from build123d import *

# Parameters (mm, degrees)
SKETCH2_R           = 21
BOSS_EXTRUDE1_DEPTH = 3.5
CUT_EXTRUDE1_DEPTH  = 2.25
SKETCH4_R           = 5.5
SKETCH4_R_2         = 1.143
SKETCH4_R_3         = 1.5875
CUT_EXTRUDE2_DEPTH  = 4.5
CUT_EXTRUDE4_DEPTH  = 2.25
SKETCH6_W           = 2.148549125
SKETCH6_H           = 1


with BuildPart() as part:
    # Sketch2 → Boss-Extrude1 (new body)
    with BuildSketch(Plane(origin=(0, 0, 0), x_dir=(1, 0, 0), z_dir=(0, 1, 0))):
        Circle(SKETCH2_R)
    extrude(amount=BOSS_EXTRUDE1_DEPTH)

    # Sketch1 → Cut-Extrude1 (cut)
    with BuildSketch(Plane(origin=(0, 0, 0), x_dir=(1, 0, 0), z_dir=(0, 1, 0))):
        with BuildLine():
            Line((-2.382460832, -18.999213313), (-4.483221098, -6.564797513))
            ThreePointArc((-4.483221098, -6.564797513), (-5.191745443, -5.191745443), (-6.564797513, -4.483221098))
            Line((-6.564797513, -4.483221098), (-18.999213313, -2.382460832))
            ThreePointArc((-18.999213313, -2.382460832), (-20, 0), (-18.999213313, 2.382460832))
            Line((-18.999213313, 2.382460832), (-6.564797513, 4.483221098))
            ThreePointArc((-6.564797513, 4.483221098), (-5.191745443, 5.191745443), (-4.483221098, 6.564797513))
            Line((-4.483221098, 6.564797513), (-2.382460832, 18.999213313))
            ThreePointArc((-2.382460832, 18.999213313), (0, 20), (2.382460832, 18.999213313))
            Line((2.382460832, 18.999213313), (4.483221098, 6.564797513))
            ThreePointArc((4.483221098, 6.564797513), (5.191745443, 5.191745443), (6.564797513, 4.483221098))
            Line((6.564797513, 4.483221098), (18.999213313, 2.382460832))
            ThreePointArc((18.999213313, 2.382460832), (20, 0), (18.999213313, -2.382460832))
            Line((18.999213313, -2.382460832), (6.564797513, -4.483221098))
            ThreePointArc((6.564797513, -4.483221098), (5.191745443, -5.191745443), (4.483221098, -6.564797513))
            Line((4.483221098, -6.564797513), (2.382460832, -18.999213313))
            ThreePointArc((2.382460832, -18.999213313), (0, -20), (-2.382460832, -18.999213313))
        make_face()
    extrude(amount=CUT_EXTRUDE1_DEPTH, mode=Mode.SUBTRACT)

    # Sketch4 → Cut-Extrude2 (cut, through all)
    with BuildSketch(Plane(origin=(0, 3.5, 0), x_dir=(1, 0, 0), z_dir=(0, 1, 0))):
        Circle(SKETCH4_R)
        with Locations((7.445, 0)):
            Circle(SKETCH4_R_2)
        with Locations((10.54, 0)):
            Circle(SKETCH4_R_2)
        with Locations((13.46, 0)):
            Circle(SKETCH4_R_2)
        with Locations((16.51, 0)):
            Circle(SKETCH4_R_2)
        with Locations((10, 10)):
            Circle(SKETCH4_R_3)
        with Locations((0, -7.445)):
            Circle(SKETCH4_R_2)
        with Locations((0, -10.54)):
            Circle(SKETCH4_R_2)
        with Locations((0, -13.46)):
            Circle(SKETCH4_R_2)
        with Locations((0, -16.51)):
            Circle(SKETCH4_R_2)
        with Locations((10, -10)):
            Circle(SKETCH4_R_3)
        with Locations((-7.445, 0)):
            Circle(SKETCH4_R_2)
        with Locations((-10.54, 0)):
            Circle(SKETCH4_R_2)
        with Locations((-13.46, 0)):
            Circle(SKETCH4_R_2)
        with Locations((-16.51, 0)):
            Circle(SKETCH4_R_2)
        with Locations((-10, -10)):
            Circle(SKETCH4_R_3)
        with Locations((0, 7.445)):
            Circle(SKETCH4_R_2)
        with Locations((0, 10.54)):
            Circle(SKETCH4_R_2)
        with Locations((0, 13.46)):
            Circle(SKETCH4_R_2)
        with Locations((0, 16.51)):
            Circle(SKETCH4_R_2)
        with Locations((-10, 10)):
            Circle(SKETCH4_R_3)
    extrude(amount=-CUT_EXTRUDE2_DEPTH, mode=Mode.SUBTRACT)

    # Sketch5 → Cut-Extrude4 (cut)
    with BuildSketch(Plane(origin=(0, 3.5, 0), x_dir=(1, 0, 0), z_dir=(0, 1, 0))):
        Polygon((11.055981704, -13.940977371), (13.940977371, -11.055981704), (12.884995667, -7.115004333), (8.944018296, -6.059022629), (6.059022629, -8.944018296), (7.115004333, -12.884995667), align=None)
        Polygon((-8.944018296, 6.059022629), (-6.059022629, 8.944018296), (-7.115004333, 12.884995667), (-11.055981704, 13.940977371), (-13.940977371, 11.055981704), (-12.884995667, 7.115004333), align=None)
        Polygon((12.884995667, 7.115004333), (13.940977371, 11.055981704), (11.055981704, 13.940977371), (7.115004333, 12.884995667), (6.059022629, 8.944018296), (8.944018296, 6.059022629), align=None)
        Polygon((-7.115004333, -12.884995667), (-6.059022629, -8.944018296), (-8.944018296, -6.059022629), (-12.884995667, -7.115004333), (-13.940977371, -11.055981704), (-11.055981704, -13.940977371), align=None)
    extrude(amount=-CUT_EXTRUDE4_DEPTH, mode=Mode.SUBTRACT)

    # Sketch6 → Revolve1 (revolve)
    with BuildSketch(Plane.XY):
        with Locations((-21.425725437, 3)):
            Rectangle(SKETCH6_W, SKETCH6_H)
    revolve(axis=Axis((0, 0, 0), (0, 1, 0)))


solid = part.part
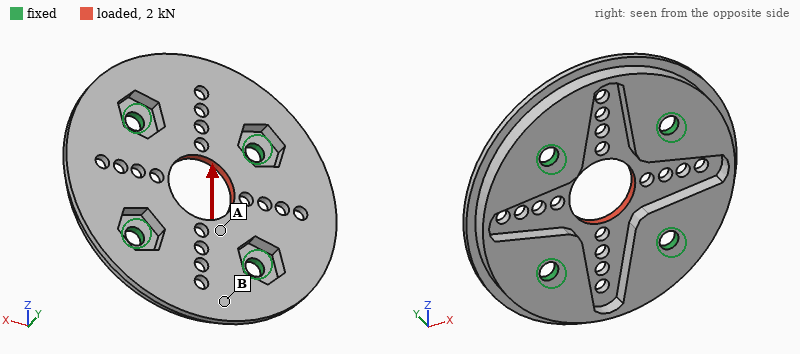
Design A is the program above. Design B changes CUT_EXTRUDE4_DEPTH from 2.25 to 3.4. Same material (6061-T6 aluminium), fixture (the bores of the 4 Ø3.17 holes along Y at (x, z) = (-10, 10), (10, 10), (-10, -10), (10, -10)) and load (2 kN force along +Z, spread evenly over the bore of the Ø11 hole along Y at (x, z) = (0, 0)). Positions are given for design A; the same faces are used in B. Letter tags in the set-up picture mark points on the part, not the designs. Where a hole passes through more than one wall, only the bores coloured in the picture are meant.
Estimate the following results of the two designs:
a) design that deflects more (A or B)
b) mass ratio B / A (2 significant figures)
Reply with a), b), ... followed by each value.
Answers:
a) B
b) 0.95
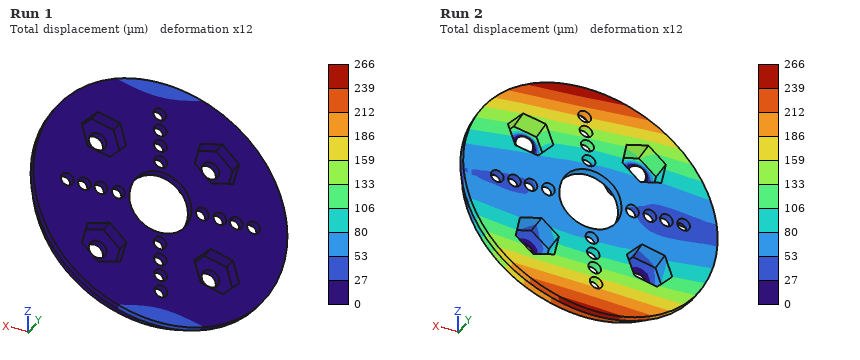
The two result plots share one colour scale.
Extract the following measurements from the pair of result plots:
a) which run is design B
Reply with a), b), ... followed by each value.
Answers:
a) Run 2
